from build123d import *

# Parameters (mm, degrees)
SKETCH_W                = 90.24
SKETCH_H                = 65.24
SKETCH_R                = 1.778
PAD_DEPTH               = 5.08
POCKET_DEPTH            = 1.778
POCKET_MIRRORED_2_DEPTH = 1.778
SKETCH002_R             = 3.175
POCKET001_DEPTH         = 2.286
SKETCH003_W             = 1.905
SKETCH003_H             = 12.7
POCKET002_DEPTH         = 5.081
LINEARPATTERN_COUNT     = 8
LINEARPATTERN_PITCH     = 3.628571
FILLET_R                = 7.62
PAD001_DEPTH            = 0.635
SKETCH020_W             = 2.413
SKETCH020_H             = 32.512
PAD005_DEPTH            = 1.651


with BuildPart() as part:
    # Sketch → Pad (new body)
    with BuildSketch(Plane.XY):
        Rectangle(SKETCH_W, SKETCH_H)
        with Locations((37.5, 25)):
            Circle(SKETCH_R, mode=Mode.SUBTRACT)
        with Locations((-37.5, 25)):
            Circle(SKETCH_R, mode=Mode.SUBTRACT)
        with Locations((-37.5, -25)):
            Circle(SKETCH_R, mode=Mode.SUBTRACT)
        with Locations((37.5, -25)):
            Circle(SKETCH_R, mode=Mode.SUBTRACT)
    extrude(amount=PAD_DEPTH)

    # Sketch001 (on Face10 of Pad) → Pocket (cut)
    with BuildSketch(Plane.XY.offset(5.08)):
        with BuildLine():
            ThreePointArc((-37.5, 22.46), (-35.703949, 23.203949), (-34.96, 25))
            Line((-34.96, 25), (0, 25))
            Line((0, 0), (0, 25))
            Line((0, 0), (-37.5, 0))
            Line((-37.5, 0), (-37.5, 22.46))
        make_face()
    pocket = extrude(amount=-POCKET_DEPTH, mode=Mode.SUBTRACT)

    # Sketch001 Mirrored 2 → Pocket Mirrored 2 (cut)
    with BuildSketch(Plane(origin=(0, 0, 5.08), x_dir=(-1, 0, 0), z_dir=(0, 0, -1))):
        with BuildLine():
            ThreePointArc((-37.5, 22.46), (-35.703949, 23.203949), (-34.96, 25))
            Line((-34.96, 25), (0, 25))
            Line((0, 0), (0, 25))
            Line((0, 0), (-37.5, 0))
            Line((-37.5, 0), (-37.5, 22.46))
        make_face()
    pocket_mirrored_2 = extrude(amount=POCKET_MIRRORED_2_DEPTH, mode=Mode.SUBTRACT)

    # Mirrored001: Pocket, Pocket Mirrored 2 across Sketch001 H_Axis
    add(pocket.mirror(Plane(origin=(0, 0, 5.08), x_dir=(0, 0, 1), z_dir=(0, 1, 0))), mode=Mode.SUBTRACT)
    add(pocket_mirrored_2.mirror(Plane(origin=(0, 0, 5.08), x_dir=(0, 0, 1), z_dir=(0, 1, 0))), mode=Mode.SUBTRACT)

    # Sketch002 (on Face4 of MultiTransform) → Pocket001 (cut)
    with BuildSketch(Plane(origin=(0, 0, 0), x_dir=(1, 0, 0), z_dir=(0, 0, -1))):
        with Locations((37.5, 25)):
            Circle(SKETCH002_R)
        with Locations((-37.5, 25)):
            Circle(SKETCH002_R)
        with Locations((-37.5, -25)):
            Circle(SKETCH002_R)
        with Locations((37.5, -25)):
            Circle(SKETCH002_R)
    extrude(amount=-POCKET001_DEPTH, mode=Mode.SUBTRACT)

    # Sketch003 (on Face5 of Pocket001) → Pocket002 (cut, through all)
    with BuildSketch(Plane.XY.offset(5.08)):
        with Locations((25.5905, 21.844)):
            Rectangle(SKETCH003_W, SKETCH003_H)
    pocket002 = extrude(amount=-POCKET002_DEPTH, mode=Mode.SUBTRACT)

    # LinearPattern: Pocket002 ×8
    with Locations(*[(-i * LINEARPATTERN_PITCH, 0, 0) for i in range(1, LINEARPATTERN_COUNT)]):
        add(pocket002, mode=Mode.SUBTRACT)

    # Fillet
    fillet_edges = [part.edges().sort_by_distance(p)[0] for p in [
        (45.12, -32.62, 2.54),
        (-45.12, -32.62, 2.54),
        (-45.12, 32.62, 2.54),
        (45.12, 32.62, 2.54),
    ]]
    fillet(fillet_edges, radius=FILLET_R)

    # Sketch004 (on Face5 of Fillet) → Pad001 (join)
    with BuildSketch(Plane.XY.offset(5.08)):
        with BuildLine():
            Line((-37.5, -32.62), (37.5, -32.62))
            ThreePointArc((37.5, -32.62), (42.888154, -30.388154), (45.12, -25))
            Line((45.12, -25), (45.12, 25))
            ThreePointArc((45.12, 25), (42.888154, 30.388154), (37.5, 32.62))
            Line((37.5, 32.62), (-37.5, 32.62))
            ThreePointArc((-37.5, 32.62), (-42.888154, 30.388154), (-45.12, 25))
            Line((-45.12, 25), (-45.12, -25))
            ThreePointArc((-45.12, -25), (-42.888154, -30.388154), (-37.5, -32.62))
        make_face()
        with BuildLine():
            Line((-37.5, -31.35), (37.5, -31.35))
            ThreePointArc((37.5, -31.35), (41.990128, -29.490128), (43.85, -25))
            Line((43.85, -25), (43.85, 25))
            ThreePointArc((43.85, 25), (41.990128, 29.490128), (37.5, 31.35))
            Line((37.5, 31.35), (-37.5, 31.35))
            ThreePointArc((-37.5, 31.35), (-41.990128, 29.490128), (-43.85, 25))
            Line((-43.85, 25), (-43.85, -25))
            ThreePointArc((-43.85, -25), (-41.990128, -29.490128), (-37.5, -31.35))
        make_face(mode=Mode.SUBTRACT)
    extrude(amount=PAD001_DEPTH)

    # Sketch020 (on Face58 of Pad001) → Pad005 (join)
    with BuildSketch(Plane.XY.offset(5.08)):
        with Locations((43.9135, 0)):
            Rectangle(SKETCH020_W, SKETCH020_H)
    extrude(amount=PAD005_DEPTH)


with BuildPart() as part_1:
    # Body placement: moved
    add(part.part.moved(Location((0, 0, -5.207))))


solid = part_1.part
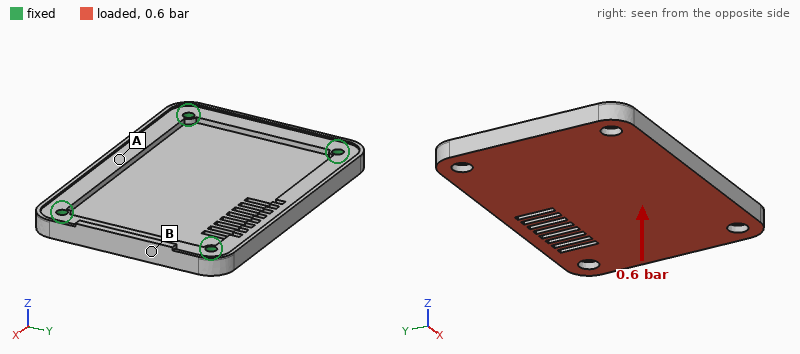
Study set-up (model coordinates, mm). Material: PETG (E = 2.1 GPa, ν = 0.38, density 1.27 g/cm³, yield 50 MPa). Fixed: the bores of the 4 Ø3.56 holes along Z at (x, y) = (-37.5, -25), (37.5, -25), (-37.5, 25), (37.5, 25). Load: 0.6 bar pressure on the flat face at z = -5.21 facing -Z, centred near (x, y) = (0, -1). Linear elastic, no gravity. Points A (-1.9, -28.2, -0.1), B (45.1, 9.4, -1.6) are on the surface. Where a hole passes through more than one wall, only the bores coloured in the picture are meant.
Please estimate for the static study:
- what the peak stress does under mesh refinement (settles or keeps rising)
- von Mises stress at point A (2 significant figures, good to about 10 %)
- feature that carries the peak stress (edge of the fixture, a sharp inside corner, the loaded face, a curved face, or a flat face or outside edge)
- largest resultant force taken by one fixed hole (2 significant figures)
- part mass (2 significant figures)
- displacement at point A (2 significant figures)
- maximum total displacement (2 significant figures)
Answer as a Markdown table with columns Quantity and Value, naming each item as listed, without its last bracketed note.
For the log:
| Quantity | Value |
|---|---|
| what the peak stress does under mesh refinement | keeps rising |
| von Mises stress at point A | 8.1 MPa |
| feature that carries the peak stress | edge of the fixture |
| largest resultant force taken by one fixed hole | 170 N |
| part mass | 28 g |
| displacement at point A | 0.64 mm |
| maximum total displacement | 0.93 mm |
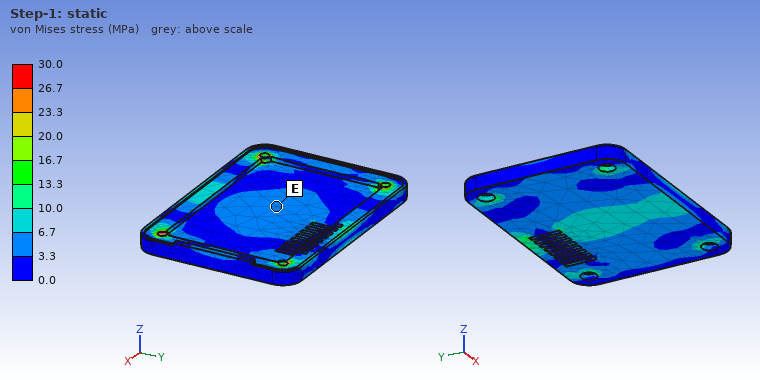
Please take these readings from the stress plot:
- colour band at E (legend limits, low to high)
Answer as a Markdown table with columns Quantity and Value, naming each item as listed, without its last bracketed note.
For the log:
| Quantity | Value |
|---|---|
| colour band at E | 3.3 to 6.7 MPa |
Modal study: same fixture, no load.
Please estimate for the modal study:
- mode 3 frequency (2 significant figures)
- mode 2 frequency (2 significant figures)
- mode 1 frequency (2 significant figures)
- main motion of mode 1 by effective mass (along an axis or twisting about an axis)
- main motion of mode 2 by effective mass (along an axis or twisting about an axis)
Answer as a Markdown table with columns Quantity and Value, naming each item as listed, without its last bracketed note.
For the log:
| Quantity | Value |
|---|---|
| mode 3 frequency | 1500 Hz |
| mode 2 frequency | 1000 Hz |
| mode 1 frequency | 720 Hz |
| main motion of mode 1 by effective mass | along Z |
| main motion of mode 2 by effective mass | twisting about X |
